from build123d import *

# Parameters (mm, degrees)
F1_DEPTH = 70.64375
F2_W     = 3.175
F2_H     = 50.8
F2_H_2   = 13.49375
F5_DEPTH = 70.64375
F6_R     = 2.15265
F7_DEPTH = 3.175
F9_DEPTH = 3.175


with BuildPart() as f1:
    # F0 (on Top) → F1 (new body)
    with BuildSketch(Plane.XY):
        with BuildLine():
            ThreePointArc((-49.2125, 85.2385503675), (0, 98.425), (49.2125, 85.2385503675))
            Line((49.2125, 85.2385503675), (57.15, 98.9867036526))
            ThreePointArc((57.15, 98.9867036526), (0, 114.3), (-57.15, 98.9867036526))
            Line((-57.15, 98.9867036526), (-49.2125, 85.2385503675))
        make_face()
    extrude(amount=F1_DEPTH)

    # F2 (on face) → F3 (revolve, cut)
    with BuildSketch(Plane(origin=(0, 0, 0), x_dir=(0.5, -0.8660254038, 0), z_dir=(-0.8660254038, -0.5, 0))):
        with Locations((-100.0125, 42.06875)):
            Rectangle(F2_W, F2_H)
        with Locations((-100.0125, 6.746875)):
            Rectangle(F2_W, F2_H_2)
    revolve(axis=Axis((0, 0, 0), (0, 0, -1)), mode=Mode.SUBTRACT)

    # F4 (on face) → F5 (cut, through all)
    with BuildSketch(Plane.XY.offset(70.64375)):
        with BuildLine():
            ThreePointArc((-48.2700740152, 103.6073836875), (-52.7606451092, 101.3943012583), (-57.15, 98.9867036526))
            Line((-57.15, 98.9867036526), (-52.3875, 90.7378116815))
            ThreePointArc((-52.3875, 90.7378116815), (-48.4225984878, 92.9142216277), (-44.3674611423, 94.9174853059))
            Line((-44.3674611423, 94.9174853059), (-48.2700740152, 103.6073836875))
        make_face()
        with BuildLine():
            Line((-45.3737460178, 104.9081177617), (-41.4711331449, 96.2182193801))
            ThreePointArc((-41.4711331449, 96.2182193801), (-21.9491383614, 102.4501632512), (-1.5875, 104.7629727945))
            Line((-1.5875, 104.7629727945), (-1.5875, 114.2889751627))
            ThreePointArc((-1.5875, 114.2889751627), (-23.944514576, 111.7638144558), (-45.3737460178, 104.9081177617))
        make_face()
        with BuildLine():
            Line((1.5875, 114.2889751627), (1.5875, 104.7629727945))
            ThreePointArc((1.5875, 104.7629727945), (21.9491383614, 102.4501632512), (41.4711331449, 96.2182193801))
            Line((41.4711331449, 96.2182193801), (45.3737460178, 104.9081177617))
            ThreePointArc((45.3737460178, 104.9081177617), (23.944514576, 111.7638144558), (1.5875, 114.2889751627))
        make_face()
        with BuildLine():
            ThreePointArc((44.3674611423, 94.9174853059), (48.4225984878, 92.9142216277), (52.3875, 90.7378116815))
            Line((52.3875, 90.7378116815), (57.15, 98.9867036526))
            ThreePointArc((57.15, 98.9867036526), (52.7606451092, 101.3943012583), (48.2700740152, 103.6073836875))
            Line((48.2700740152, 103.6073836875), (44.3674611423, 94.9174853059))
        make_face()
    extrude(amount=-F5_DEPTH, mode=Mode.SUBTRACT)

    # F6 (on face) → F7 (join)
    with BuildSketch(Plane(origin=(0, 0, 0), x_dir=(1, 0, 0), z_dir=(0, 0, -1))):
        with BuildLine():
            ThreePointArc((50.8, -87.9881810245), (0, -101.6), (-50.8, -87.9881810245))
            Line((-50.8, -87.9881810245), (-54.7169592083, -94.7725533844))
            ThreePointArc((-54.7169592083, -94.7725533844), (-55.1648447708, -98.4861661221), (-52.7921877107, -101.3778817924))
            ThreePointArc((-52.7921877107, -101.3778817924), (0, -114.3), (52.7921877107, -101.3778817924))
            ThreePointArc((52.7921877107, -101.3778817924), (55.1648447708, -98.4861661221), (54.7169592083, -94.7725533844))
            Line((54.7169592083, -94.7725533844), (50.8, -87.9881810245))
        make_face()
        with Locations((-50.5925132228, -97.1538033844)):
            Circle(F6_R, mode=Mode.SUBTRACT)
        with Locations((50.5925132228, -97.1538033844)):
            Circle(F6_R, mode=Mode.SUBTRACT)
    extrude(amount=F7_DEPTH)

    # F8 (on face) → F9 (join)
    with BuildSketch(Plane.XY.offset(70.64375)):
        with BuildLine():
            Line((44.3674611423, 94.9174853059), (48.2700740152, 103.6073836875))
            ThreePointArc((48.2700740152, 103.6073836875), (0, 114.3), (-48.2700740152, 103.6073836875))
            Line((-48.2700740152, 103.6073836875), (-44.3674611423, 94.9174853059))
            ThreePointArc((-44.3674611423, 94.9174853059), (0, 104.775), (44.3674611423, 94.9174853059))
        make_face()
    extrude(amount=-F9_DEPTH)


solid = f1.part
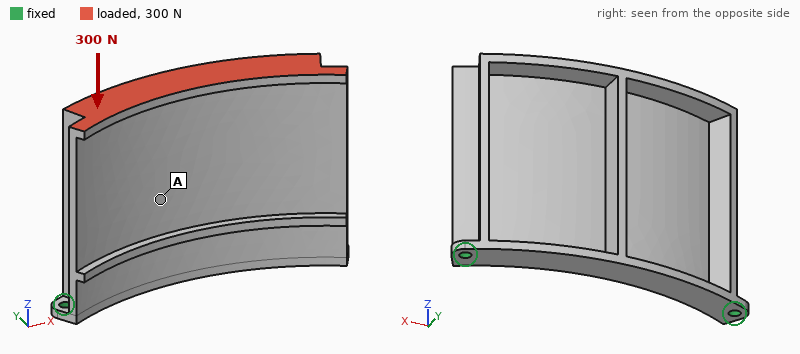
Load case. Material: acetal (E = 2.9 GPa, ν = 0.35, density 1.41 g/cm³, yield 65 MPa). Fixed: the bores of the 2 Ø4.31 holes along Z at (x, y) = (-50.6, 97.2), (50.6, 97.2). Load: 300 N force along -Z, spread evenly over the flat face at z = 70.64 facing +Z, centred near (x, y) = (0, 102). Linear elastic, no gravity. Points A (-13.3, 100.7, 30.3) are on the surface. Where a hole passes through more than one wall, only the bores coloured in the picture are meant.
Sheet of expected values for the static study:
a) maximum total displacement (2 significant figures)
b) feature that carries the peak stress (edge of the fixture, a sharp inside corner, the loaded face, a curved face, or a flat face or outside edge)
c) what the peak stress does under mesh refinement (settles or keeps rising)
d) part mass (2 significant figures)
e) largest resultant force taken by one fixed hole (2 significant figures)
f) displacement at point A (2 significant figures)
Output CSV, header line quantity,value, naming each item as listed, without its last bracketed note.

quantity,value
maximum total displacement,1.4 mm
feature that carries the peak stress,edge of the fixture
what the peak stress does under mesh refinement,keeps rising
part mass,56 g
largest resultant force taken by one fixed hole,170 N
displacement at point A,0.59 mm
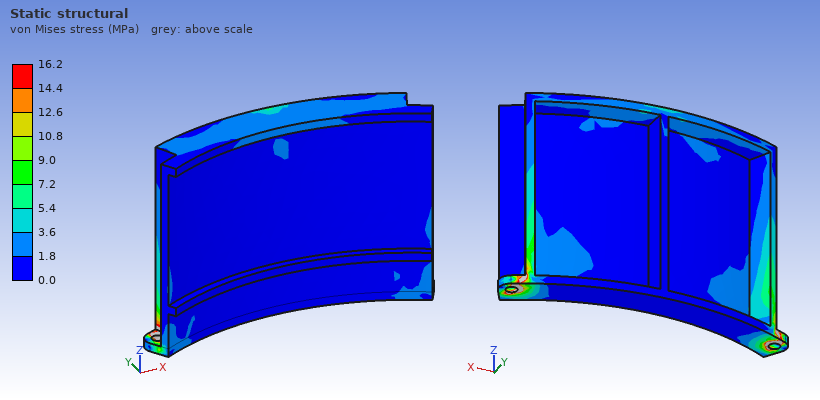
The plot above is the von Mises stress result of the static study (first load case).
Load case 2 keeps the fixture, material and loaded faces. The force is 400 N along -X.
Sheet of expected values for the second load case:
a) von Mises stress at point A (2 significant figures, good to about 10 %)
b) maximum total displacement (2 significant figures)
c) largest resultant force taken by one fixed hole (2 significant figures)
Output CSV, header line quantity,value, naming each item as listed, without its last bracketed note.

quantity,value
von Mises stress at point A,3.2 MPa
maximum total displacement,0.53 mm
largest resultant force taken by one fixed hole,360 N
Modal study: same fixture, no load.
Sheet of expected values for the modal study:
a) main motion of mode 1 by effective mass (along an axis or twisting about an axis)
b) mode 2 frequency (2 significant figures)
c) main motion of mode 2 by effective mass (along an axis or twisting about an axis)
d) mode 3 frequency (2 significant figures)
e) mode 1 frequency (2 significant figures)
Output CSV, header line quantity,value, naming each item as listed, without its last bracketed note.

quantity,value
main motion of mode 1 by effective mass,along Y
mode 2 frequency,300 Hz
main motion of mode 2 by effective mass,twisting about Z
mode 3 frequency,1000 Hz
mode 1 frequency,160 Hz
